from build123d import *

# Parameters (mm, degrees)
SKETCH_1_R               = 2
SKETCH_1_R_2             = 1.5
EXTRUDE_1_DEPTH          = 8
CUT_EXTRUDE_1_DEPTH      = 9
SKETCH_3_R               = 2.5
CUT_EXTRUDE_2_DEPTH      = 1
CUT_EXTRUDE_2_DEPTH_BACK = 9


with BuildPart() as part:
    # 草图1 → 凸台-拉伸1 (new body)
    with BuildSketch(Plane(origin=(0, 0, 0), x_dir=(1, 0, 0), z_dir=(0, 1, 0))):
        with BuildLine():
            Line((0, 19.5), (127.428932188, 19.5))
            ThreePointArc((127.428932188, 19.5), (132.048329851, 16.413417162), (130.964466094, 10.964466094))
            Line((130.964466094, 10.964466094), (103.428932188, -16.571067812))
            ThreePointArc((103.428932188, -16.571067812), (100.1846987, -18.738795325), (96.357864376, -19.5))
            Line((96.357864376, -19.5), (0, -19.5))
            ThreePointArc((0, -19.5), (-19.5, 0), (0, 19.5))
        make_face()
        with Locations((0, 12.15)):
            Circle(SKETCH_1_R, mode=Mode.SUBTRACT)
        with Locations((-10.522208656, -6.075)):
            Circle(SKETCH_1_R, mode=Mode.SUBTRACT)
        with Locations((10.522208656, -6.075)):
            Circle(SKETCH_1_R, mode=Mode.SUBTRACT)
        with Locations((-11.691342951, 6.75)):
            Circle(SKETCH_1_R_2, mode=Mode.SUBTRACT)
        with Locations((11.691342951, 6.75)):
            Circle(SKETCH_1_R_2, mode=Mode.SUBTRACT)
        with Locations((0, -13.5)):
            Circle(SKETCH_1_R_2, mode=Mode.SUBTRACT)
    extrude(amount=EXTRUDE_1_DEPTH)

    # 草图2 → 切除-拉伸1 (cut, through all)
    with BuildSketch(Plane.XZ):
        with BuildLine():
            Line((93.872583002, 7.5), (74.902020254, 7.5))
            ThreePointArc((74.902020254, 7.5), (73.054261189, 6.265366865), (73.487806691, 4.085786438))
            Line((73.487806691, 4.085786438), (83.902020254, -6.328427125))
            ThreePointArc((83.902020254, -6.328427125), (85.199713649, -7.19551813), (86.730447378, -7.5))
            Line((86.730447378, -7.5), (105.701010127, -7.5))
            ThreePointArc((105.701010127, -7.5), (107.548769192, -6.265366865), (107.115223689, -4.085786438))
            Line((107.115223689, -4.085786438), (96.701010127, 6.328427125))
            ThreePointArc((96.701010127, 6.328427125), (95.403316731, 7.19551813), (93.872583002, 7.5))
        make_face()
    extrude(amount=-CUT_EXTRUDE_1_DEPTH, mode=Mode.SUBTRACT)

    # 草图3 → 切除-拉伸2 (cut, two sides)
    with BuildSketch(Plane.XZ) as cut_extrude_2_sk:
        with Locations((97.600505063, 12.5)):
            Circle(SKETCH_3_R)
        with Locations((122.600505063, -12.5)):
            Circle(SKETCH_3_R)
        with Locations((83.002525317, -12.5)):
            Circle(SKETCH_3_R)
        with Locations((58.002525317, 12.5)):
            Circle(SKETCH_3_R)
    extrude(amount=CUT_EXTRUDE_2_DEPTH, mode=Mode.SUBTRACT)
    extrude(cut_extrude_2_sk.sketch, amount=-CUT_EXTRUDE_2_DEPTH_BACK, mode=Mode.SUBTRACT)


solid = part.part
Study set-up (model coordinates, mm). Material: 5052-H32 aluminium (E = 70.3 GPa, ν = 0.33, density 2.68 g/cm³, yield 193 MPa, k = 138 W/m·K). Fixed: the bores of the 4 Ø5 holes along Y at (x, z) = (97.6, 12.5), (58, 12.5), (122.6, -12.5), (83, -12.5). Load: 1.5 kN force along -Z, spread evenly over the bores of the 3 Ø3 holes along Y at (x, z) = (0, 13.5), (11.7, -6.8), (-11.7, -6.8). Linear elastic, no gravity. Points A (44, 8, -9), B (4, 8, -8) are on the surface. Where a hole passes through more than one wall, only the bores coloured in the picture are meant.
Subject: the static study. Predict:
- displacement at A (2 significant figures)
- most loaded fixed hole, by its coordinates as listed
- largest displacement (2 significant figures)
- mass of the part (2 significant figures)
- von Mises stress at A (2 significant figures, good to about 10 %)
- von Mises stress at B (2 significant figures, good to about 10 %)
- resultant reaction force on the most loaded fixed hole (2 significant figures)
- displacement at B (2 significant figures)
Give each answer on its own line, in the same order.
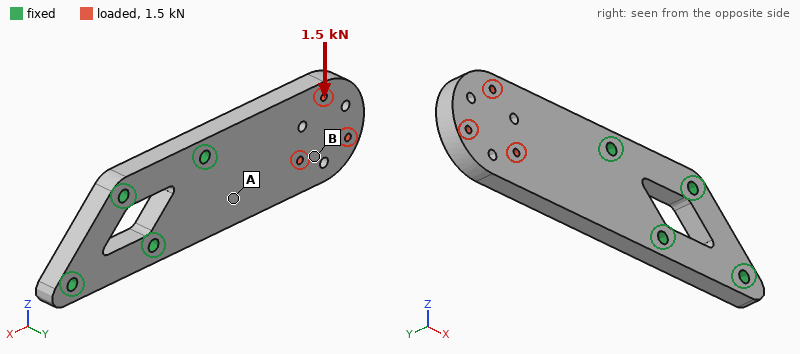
16 µm
(58, 12.5)
95 µm
100 g
17 MPa
7.8 MPa
3.3 kN
64 µm
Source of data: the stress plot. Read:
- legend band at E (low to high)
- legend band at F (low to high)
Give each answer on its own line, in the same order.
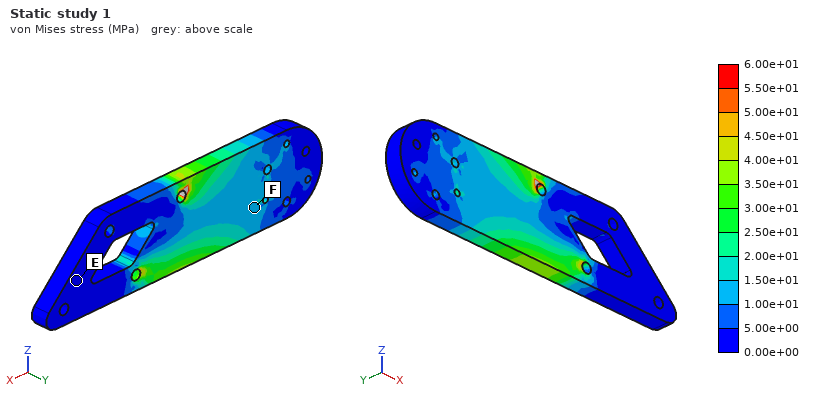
0.00e+00 to 5.00e+00 MPa
1.00e+01 to 1.50e+01 MPa
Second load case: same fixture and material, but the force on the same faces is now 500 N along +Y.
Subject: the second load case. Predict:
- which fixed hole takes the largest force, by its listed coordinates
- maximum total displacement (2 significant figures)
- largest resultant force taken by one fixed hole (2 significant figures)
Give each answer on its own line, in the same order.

(58, 12.5)
0.51 mm
890 N
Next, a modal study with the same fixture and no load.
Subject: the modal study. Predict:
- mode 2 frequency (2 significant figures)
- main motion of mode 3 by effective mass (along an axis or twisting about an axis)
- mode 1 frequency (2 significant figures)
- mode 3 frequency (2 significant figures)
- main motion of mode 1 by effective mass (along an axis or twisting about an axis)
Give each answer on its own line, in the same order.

4000 Hz
along Z
1100 Hz
4100 Hz
along Y
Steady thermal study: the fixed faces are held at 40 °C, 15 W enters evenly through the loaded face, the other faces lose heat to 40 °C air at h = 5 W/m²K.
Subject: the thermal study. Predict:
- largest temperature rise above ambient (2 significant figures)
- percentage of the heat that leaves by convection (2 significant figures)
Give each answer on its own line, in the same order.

24 K
3.6 %
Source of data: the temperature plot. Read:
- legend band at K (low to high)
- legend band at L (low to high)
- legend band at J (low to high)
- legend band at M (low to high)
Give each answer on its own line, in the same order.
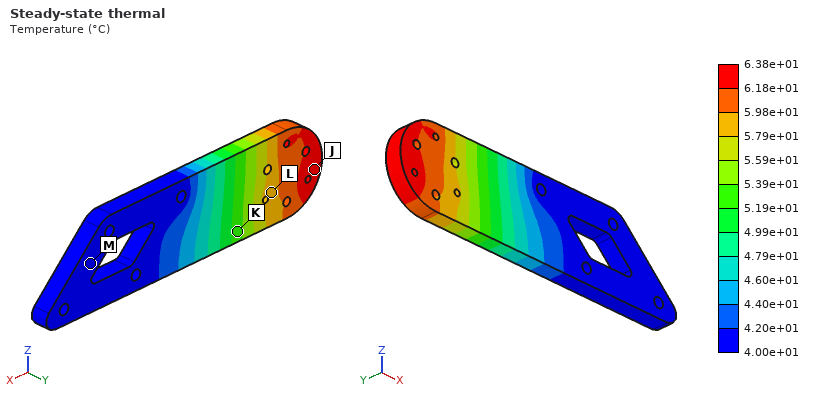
5.19e+01 to 5.39e+01 °C
5.79e+01 to 5.98e+01 °C
6.18e+01 to 6.38e+01 °C
4.00e+01 to 4.20e+01 °C
